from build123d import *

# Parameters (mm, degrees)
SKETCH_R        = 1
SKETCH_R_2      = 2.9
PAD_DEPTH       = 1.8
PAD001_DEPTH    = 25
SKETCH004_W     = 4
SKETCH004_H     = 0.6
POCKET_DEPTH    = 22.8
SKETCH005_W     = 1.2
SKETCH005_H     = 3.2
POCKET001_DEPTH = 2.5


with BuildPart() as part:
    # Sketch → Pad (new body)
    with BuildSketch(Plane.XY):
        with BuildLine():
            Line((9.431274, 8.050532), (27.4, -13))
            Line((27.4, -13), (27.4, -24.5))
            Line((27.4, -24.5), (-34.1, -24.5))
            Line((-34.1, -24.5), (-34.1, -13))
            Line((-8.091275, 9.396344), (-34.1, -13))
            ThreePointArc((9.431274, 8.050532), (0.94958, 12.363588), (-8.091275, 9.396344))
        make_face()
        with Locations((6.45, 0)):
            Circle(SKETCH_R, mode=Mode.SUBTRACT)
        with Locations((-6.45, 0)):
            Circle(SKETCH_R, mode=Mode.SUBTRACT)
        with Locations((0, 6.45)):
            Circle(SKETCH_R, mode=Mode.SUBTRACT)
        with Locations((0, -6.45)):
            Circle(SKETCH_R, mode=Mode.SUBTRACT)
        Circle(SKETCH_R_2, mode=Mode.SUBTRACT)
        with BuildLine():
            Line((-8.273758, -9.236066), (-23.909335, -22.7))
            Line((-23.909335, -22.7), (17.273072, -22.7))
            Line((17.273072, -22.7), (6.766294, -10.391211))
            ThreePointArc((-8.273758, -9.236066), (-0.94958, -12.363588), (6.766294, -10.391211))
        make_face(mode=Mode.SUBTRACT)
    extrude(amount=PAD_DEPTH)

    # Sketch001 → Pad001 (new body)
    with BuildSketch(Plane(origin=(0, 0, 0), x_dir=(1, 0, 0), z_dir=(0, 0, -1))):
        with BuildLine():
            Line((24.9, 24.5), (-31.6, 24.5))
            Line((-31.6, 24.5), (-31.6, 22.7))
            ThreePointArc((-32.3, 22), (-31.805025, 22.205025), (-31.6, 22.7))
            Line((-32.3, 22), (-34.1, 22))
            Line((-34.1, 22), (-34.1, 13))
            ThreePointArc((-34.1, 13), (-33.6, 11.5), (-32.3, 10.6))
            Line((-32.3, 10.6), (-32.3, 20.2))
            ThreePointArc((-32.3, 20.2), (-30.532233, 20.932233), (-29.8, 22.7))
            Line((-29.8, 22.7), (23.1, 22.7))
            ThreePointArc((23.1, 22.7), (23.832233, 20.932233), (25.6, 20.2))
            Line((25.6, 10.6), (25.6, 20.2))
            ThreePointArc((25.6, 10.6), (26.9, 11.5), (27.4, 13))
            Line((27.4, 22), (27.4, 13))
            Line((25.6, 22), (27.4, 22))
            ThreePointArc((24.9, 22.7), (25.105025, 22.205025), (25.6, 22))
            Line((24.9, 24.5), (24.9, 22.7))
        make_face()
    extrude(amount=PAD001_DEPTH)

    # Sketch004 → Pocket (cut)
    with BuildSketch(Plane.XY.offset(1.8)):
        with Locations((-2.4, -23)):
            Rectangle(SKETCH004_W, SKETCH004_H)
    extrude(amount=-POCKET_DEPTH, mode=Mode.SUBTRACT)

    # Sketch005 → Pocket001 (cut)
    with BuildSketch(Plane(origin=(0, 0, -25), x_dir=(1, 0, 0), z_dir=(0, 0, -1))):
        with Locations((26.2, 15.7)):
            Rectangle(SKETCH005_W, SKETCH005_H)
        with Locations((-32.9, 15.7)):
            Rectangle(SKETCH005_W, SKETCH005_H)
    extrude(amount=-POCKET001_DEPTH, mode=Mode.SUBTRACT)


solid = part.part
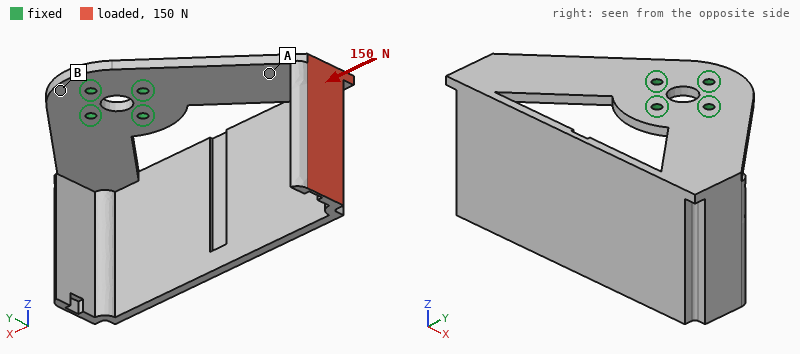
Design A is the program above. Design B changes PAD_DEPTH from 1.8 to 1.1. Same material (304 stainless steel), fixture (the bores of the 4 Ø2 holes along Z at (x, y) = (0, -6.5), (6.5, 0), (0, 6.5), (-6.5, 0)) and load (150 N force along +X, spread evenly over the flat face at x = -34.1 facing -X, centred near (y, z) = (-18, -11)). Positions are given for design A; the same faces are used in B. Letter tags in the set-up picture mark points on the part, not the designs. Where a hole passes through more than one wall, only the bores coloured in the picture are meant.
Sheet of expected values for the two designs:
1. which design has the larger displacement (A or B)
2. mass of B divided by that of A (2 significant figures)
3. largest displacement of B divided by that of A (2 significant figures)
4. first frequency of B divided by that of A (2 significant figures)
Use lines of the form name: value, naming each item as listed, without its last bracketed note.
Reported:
which design has the larger displacement: B
mass of B divided by that of A: 0.85
largest displacement of B divided by that of A: 2.9
first frequency of B divided by that of A: 0.51
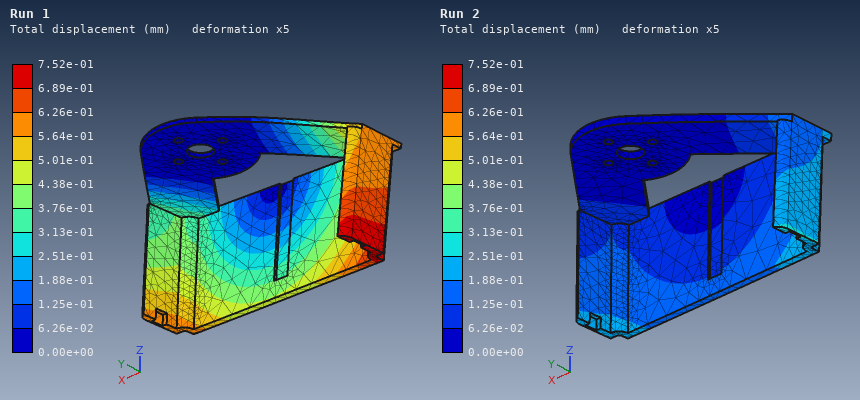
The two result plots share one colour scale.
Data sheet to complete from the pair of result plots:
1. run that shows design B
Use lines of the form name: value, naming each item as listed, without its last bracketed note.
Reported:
run that shows design B: Run 1
